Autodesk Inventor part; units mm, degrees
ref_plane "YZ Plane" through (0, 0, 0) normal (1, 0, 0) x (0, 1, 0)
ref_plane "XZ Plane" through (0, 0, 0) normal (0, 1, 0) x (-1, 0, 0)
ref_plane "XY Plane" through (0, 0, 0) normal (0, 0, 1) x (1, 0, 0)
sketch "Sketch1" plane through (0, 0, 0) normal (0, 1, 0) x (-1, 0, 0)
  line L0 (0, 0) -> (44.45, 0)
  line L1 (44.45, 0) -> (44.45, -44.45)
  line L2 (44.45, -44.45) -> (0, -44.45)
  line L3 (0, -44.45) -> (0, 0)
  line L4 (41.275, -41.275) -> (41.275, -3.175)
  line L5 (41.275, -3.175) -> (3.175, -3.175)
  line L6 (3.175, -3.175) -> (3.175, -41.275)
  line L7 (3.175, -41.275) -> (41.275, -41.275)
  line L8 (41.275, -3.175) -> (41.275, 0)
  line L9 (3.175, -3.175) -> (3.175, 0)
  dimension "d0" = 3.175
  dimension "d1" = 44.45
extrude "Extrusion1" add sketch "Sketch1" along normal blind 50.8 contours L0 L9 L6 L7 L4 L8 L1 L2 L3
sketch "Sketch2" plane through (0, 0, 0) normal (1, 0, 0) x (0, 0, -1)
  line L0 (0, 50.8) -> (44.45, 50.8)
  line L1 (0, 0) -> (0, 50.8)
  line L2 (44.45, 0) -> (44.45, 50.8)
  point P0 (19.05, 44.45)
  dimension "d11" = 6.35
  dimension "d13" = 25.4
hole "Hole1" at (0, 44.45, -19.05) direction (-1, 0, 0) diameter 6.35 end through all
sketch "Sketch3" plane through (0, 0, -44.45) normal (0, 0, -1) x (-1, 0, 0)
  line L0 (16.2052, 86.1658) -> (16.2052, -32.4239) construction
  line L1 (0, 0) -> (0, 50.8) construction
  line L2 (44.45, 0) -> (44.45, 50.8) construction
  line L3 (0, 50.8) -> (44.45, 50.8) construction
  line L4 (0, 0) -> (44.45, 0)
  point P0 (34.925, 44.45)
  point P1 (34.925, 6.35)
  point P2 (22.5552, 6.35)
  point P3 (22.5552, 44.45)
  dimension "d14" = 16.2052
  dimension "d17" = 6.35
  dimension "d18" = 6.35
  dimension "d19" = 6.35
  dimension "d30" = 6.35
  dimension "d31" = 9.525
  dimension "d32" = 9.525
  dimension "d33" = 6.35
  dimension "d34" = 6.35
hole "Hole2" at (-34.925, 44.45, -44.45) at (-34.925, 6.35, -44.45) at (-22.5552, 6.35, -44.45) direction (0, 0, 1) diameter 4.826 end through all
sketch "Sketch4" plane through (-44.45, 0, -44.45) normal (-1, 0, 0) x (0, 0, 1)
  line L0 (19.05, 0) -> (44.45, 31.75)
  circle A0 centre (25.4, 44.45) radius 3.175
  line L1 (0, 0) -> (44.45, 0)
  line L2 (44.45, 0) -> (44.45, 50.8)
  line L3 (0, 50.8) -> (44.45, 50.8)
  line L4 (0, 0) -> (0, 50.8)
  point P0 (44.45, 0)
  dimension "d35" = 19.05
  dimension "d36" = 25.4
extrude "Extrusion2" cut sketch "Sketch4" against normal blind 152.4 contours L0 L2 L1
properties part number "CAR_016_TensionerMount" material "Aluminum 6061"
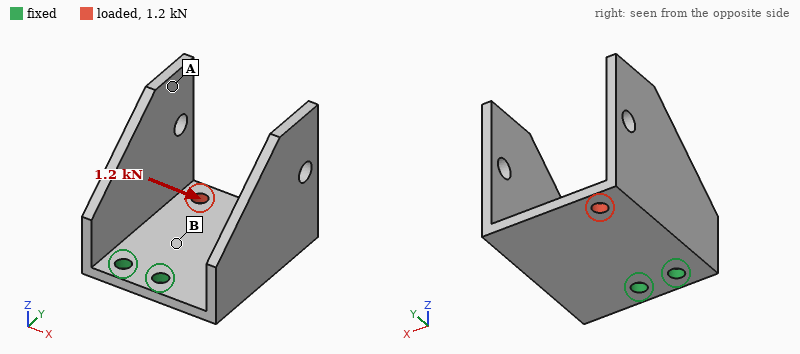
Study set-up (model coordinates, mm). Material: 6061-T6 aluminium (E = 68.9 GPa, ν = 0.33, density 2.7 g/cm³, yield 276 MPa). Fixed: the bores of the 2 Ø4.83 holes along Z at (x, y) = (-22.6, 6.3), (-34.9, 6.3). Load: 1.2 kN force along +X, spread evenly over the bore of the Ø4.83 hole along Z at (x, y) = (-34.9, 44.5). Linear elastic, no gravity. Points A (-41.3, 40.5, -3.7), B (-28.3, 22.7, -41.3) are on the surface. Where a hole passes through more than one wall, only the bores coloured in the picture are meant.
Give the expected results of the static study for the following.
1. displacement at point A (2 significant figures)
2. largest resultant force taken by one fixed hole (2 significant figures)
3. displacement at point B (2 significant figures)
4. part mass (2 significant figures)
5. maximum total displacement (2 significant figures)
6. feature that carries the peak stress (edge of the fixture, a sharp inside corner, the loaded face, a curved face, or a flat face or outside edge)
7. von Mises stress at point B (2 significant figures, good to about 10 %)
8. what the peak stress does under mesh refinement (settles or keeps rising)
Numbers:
0.063 mm
2.7 kN
0.027 mm
47 g
0.10 mm
edge of the fixture
35 MPa
keeps rising
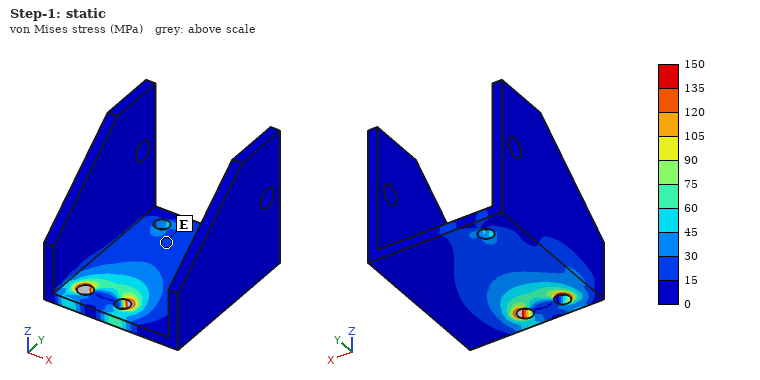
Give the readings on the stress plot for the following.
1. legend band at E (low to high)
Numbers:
15 to 30 MPa
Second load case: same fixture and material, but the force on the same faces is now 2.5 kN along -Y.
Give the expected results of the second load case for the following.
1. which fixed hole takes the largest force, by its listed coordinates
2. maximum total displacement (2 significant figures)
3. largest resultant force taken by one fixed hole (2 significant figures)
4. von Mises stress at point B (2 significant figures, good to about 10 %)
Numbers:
(-34.9, 6.3)
38 µm
2.2 kN
25 MPa
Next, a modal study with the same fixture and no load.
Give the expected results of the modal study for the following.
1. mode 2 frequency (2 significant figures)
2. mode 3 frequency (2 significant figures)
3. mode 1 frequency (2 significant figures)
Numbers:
1000 Hz
1200 Hz
730 Hz
